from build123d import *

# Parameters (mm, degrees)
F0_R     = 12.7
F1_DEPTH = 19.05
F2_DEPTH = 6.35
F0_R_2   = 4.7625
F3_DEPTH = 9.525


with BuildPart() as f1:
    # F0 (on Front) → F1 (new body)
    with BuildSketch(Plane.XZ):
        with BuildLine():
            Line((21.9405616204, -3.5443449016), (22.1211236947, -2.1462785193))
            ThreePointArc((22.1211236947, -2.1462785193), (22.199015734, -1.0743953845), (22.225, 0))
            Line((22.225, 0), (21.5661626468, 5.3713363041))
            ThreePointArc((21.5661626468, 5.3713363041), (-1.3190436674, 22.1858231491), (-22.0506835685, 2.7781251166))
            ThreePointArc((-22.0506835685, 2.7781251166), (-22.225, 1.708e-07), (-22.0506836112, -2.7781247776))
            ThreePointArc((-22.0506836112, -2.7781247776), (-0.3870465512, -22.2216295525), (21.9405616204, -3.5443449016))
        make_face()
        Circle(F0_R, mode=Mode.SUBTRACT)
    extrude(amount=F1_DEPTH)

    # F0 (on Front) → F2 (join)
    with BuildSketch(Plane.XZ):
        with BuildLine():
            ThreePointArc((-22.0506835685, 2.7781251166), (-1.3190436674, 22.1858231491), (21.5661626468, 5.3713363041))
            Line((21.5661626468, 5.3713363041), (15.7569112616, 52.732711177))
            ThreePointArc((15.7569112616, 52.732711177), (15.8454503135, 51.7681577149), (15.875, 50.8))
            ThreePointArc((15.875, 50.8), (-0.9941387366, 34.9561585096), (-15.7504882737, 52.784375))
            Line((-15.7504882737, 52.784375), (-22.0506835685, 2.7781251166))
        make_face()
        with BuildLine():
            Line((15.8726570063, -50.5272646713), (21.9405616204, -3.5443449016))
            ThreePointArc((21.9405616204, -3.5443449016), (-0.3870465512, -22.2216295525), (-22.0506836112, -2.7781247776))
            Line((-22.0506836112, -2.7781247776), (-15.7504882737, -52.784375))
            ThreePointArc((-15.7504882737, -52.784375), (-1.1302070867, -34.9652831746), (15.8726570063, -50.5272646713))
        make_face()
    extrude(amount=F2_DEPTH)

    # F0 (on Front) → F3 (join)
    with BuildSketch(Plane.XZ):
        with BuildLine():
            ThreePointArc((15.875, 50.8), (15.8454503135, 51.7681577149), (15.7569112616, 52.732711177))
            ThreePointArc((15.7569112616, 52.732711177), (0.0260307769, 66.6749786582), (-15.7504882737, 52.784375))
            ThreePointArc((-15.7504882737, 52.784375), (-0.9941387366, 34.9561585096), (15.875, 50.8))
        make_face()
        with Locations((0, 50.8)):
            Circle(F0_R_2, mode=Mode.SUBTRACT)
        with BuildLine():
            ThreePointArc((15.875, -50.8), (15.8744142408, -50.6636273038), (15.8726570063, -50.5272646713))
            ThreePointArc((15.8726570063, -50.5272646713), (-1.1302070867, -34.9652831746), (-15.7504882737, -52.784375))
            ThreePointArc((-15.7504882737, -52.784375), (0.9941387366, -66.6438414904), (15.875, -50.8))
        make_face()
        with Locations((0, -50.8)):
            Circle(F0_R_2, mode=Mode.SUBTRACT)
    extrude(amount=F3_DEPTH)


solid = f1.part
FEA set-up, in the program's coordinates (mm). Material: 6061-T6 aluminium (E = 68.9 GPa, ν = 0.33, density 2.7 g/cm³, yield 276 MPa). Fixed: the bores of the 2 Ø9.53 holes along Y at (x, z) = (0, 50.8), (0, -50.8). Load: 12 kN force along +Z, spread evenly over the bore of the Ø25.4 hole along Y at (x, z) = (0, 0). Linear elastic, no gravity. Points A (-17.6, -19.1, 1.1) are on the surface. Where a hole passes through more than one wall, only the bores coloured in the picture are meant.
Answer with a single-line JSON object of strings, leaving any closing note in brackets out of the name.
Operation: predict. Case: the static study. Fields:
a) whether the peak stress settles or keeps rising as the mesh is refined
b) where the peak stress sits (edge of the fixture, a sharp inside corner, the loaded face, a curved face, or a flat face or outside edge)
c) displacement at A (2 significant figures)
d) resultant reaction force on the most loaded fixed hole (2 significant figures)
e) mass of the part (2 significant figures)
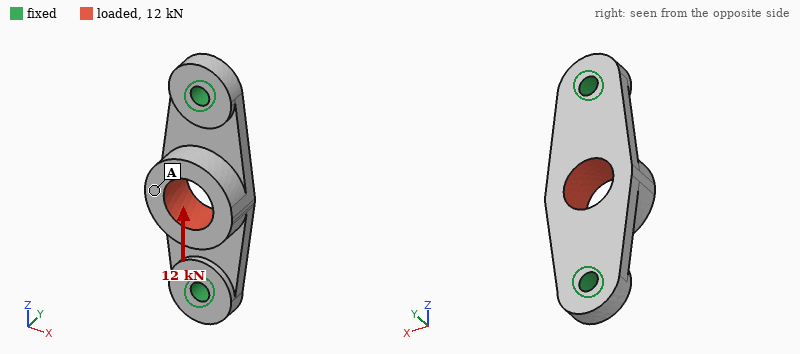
{"whether the peak stress settles or keeps rising as the mesh is refined": "keeps rising", "where the peak stress sits": "edge of the fixture", "displacement at A": "37 µm", "resultant reaction force on the most loaded fixed hole": "6.1 kN", "mass of the part": "120 g"}
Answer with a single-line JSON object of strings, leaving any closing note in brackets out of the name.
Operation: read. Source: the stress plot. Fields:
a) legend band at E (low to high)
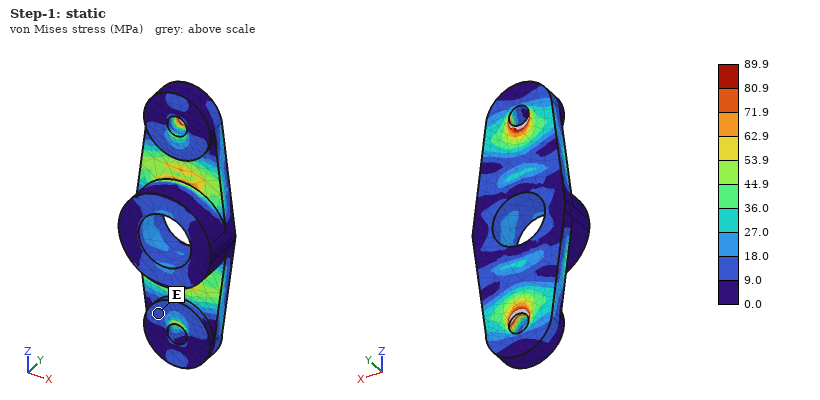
{"legend band at E": "9.0 to 18.0 MPa"}
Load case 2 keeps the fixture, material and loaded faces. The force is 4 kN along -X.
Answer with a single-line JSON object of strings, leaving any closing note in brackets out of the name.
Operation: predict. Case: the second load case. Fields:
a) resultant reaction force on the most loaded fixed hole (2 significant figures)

{"resultant reaction force on the most loaded fixed hole": "2.0 kN"}
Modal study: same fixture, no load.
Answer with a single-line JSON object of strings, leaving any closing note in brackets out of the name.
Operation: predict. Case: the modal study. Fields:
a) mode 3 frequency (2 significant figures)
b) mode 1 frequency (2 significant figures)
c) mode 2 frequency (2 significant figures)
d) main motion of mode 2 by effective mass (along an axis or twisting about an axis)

{"mode 3 frequency": "8500 Hz", "mode 1 frequency": "3800 Hz", "mode 2 frequency": "4200 Hz", "main motion of mode 2 by effective mass": "along Y"}
